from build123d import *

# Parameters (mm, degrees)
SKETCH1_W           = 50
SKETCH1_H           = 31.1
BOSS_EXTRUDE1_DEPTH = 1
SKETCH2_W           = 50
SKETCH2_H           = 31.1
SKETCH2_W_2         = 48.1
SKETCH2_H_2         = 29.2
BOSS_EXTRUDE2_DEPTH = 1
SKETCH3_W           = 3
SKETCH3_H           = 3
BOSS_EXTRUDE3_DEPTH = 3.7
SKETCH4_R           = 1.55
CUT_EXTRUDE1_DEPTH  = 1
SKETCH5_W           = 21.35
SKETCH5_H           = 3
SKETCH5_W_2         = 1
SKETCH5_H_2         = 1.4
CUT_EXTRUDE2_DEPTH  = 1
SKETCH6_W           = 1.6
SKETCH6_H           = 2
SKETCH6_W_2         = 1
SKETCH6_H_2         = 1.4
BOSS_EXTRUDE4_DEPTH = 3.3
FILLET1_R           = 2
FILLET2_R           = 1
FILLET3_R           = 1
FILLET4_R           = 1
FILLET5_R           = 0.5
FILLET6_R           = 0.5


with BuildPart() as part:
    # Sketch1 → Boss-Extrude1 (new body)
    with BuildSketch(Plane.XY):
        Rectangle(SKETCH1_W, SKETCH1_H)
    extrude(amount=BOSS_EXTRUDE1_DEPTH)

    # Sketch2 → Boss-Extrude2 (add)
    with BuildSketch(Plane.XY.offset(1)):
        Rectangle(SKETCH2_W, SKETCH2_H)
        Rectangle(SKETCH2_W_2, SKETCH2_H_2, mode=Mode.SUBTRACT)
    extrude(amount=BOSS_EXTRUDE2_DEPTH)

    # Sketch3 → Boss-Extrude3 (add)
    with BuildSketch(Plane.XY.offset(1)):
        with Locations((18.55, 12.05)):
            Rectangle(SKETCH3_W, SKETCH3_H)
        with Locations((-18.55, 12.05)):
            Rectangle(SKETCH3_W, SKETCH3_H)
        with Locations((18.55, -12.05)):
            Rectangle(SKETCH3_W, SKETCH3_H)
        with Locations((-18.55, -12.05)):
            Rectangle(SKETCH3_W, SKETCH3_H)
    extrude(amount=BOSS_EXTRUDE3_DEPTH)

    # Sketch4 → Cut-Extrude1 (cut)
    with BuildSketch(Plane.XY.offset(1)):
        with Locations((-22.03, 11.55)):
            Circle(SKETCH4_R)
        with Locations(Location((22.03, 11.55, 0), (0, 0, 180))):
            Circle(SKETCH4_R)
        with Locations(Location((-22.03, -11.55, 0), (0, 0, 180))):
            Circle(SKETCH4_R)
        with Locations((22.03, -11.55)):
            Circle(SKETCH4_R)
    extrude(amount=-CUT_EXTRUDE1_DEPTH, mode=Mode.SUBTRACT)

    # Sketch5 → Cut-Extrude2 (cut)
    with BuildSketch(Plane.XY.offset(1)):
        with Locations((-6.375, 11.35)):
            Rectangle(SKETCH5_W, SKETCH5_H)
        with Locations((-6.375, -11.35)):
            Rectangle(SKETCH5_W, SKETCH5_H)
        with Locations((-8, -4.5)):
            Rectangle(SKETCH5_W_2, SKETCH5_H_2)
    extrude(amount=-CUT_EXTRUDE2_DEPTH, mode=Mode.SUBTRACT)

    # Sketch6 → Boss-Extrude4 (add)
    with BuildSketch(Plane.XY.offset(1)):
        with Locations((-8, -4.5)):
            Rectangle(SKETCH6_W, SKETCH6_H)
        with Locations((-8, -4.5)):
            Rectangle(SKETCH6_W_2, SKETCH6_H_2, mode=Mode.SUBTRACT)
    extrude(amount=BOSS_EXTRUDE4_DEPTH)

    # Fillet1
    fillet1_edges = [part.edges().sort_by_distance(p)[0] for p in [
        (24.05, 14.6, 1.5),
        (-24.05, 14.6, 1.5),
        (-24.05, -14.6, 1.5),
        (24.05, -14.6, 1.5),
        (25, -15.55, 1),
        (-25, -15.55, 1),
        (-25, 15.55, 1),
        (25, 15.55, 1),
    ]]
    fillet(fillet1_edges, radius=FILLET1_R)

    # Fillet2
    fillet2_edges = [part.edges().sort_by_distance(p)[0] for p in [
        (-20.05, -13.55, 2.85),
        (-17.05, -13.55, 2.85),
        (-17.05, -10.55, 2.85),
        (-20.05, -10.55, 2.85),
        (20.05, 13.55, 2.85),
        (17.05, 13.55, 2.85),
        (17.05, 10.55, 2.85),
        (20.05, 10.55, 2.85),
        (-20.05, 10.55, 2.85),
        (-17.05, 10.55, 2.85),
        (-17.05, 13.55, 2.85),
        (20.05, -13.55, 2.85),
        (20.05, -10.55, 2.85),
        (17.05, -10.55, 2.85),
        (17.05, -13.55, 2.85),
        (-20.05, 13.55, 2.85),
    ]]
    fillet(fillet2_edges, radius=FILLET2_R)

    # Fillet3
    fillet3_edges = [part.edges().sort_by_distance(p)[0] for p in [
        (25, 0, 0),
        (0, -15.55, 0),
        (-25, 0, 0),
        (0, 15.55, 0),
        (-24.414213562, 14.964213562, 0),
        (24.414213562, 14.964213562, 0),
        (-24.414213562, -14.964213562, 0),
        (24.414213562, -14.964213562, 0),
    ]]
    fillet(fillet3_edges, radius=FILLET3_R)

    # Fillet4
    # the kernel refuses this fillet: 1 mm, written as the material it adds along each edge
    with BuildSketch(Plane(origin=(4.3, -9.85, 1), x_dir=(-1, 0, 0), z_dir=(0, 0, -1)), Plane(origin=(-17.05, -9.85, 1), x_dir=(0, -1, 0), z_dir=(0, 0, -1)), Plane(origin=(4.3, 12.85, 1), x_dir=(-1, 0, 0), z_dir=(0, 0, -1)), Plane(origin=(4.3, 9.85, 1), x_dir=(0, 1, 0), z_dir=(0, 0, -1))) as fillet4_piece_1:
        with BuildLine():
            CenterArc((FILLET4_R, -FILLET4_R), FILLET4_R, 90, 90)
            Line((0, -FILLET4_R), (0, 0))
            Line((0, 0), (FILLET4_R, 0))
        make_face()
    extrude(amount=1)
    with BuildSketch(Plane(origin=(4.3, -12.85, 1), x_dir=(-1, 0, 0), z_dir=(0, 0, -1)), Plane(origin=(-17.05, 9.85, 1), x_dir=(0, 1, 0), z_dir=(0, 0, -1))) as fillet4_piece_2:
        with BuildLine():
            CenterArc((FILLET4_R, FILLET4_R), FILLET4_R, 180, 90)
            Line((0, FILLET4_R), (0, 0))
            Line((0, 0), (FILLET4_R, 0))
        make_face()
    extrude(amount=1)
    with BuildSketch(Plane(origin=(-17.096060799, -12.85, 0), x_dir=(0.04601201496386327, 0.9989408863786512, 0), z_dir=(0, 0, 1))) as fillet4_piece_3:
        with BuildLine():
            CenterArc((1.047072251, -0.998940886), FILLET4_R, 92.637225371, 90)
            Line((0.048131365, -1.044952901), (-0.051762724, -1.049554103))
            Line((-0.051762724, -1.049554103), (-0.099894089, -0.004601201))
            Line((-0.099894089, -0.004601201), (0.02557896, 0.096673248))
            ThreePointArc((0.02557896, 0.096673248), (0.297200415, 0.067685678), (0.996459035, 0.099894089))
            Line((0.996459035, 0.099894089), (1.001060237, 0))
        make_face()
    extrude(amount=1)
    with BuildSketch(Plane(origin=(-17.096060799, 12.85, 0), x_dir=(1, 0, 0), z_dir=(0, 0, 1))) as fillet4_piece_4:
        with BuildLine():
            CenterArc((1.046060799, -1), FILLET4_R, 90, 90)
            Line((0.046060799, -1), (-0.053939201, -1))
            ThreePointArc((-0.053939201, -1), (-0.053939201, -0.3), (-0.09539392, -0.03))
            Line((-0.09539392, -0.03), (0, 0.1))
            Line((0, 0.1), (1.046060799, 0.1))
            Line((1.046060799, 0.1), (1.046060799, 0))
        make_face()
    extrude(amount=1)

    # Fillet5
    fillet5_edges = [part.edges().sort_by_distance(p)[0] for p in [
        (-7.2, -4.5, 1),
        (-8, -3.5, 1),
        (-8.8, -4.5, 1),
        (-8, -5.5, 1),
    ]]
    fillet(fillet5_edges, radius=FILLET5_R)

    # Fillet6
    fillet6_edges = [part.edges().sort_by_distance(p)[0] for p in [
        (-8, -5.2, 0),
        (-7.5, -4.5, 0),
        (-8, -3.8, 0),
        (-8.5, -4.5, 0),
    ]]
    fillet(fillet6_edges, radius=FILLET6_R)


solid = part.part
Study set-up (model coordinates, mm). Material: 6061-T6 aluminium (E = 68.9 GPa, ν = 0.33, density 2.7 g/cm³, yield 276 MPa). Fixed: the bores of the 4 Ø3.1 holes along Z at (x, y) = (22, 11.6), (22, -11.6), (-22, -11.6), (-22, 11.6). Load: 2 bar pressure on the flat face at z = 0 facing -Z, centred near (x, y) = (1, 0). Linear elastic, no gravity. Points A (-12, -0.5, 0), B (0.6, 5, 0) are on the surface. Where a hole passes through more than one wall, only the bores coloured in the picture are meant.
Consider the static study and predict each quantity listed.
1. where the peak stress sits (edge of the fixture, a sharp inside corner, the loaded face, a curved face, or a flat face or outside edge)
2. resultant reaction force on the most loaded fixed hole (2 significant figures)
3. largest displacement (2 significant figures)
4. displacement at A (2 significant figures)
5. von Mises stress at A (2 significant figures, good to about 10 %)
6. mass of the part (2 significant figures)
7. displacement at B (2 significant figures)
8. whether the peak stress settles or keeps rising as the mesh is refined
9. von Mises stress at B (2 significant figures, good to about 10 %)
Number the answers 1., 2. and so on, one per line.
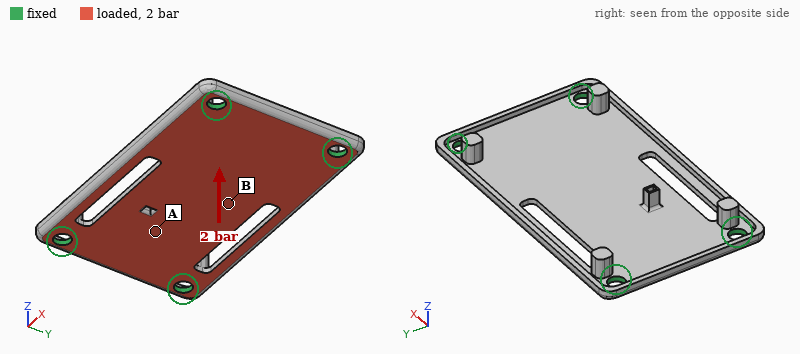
1. edge of the fixture
2. 67 N
3. 0.25 mm
4. 0.15 mm
5. 31 MPa
6. 4.4 g
7. 0.24 mm
8. keeps rising
9. 63 MPa
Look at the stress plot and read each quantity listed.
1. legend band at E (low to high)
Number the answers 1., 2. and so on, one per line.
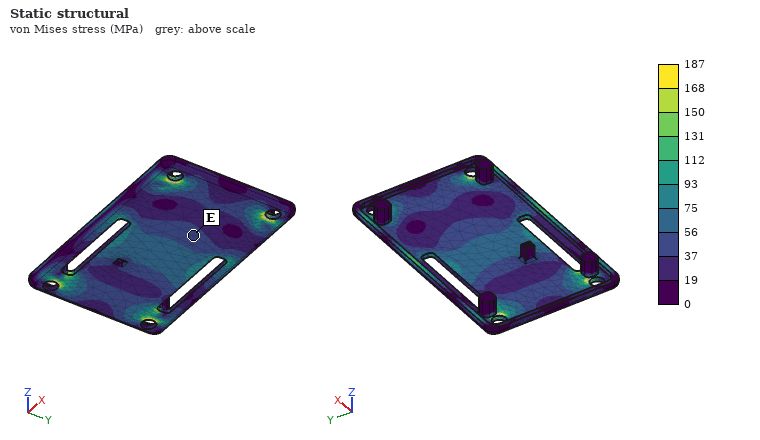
1. 37 to 56 MPa
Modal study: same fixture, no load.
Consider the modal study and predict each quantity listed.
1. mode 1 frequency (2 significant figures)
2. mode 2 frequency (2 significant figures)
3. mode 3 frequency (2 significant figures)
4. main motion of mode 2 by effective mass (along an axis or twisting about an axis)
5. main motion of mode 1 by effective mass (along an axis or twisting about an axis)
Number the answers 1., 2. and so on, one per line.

1. 3200 Hz
2. 5000 Hz
3. 6600 Hz
4. twisting about X
5. along Z
